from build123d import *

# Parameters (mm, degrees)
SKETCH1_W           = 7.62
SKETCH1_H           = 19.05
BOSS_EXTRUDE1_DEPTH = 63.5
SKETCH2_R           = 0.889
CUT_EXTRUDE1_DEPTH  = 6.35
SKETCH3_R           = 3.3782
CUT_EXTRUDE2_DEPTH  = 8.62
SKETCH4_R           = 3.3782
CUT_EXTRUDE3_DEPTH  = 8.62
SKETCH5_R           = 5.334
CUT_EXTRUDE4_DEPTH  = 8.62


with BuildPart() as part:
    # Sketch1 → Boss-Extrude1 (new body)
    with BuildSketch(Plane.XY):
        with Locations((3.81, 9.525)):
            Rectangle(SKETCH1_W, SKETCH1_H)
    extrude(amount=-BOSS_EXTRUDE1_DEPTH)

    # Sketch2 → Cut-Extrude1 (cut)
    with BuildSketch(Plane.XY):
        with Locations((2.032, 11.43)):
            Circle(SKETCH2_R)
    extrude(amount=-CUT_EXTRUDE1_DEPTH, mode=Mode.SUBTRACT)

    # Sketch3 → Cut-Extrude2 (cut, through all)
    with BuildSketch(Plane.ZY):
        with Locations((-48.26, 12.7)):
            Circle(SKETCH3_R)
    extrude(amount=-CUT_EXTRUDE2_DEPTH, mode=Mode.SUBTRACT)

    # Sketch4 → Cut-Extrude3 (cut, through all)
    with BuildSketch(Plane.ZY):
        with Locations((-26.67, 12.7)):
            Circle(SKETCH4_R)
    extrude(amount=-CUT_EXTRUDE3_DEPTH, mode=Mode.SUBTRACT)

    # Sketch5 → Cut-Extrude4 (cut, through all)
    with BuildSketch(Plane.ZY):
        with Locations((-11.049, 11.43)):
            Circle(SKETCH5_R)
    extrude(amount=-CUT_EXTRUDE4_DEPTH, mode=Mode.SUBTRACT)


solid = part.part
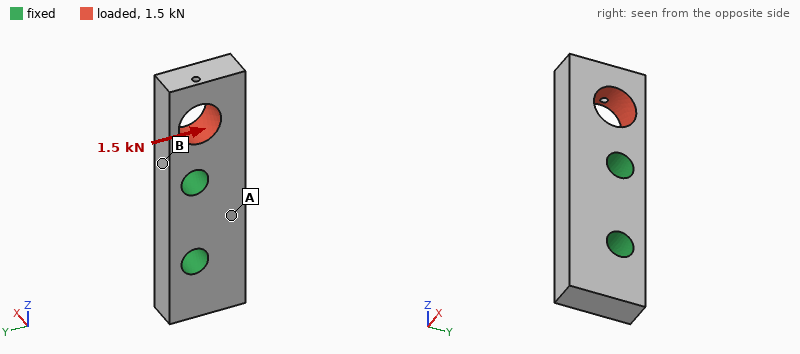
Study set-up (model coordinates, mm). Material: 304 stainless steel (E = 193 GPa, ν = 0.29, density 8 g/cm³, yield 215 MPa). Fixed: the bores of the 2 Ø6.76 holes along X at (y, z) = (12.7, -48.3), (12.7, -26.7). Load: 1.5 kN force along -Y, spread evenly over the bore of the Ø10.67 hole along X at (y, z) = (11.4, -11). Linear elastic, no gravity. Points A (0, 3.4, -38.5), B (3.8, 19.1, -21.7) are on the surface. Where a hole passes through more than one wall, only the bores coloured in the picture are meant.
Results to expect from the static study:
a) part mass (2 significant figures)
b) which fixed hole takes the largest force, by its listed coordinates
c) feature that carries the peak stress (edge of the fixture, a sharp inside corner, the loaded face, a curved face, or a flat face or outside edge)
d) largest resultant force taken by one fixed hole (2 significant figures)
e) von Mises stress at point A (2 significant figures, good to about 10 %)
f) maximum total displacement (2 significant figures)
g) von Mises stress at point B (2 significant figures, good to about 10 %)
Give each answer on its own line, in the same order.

64 g
(12.7, -26.7)
edge of the fixture
2.0 kN
11 MPa
16 µm
47 MPa
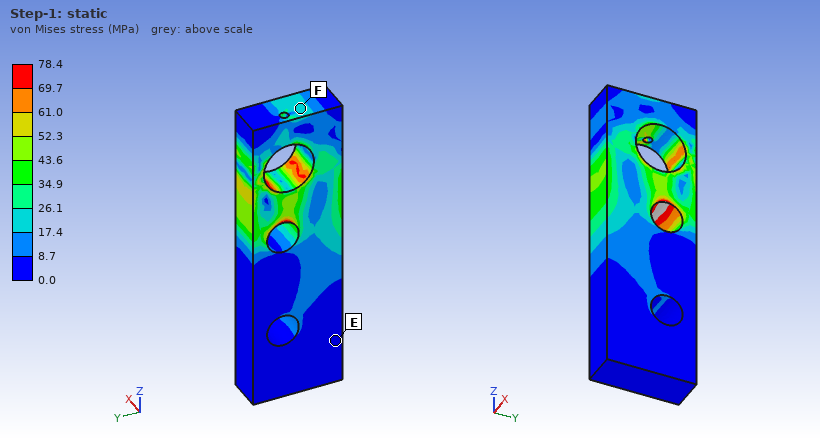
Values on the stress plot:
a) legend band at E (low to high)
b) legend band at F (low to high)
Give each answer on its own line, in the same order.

0.0 to 8.7 MPa
17.4 to 26.1 MPa
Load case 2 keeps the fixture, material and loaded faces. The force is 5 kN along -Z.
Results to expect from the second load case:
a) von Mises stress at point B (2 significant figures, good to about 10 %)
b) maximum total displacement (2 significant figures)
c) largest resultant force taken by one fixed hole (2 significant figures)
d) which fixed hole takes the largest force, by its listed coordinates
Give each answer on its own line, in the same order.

58 MPa
9.1 µm
4.5 kN
(12.7, -26.7)
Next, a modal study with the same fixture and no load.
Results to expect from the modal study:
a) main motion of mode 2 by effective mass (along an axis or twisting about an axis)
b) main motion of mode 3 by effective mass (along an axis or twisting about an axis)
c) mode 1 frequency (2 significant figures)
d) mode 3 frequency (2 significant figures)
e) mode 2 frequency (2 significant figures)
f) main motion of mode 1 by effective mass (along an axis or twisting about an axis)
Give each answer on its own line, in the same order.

along Y
twisting about Z
8200 Hz
17 kHz
12 kHz
along X
